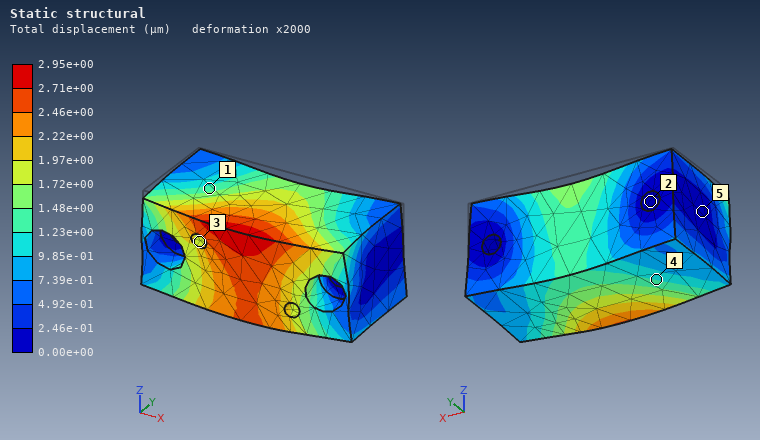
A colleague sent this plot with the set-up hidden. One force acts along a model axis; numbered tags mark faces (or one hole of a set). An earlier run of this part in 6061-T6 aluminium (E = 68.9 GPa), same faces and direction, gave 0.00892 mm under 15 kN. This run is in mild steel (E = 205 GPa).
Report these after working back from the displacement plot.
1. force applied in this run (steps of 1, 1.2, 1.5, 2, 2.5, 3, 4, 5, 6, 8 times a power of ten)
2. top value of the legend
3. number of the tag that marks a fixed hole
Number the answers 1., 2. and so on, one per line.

1. 15 kN
2. 2.95e+00 µm
3. 2
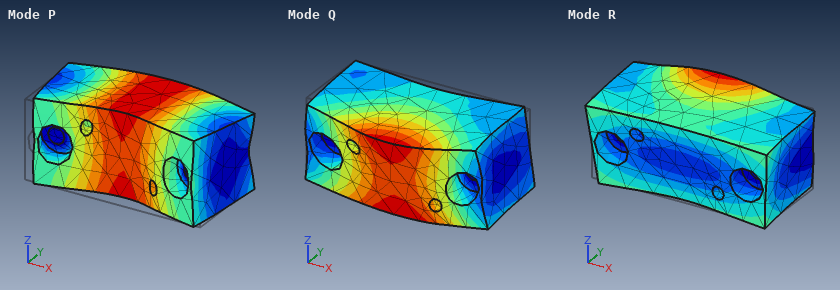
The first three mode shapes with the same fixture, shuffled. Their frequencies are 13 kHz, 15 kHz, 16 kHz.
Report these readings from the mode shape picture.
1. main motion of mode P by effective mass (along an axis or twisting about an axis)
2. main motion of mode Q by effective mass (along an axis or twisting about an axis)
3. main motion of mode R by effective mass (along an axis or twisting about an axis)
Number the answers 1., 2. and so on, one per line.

1. along Y
2. along Z
3. along Z
